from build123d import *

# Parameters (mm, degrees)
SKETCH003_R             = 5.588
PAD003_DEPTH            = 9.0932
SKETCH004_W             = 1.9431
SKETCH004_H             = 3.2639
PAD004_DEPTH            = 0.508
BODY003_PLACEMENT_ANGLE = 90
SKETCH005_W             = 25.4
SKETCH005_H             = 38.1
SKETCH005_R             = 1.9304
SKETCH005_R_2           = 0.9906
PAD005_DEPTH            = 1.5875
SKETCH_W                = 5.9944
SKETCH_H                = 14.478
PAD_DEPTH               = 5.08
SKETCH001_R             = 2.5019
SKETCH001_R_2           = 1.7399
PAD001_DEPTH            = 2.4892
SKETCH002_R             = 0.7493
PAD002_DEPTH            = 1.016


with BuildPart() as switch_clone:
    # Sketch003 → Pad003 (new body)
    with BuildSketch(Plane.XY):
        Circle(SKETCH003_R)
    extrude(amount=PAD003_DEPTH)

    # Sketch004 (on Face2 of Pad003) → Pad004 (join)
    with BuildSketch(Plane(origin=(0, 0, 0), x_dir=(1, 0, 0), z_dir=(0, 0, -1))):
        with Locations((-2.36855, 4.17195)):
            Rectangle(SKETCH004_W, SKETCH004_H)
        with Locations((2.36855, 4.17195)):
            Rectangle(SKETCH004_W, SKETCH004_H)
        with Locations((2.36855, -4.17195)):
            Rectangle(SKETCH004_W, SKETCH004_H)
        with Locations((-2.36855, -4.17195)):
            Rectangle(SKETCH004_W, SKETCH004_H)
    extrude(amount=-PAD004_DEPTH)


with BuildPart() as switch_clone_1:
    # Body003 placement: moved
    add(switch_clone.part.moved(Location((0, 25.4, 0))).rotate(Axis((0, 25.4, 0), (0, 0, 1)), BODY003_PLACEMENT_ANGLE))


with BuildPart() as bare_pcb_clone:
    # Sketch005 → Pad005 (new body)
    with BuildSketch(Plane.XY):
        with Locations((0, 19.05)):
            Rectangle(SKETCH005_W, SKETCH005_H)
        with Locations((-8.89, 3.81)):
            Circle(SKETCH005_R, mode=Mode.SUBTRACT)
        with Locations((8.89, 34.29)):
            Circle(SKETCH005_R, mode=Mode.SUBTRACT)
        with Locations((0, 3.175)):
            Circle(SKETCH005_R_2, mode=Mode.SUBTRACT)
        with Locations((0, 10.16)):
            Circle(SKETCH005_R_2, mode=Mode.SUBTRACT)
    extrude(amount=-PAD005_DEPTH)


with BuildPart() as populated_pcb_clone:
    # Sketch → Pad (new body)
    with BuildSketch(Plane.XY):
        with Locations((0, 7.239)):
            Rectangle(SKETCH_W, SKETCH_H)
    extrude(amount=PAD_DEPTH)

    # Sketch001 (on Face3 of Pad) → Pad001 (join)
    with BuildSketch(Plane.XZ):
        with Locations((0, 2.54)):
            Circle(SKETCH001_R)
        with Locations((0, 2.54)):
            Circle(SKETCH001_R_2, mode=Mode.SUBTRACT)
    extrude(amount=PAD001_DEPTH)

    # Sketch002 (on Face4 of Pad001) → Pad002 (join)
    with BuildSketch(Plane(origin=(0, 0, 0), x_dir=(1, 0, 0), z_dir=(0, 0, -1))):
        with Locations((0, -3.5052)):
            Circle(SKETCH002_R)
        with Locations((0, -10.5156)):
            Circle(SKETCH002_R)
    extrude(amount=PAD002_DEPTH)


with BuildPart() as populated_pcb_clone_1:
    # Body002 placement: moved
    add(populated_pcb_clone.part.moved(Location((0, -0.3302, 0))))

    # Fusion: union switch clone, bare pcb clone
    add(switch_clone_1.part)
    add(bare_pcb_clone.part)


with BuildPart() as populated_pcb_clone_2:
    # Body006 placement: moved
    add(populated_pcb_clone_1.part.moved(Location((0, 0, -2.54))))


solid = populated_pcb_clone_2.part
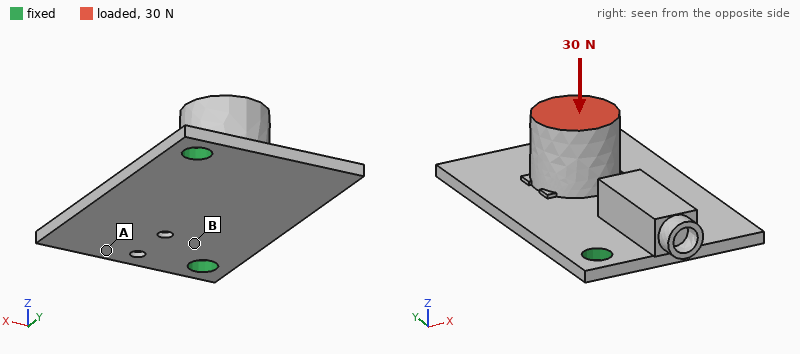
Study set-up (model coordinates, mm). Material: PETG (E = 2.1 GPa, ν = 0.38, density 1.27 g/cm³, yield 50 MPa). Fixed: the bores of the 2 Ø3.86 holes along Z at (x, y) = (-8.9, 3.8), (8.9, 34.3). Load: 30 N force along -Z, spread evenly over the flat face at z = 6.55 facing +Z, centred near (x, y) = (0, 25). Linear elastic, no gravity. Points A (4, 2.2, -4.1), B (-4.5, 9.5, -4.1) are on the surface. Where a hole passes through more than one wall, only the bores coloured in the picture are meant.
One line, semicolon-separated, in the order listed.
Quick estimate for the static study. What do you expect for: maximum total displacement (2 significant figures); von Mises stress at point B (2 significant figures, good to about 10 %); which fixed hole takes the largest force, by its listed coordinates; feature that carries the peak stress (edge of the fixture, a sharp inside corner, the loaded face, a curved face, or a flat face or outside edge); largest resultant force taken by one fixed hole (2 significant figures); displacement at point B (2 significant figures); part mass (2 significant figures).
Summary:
0.47 mm; 3.6 MPa; (8.9, 34.3); a flat face or outside edge; 21 N; 0.082 mm; 3.6 g
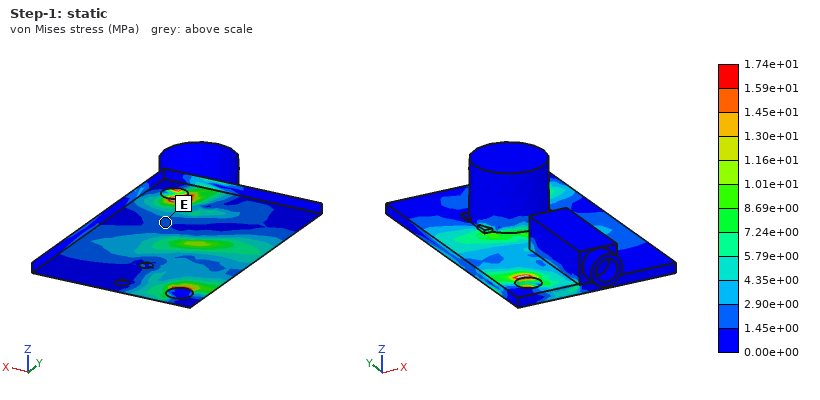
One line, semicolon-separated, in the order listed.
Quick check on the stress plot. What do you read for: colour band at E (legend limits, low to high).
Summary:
1.45e+00 to 2.90e+00 MPa
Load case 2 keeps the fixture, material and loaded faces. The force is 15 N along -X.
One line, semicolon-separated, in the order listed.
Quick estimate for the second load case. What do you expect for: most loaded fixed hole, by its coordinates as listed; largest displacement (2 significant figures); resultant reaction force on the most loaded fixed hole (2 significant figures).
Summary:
(8.9, 34.3); 0.56 mm; 11 N
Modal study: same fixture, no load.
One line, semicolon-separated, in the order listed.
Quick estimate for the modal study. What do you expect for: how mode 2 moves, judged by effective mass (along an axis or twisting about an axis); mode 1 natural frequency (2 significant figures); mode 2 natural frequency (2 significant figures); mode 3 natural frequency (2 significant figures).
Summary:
along Z; 830 Hz; 1100 Hz; 1900 Hz
